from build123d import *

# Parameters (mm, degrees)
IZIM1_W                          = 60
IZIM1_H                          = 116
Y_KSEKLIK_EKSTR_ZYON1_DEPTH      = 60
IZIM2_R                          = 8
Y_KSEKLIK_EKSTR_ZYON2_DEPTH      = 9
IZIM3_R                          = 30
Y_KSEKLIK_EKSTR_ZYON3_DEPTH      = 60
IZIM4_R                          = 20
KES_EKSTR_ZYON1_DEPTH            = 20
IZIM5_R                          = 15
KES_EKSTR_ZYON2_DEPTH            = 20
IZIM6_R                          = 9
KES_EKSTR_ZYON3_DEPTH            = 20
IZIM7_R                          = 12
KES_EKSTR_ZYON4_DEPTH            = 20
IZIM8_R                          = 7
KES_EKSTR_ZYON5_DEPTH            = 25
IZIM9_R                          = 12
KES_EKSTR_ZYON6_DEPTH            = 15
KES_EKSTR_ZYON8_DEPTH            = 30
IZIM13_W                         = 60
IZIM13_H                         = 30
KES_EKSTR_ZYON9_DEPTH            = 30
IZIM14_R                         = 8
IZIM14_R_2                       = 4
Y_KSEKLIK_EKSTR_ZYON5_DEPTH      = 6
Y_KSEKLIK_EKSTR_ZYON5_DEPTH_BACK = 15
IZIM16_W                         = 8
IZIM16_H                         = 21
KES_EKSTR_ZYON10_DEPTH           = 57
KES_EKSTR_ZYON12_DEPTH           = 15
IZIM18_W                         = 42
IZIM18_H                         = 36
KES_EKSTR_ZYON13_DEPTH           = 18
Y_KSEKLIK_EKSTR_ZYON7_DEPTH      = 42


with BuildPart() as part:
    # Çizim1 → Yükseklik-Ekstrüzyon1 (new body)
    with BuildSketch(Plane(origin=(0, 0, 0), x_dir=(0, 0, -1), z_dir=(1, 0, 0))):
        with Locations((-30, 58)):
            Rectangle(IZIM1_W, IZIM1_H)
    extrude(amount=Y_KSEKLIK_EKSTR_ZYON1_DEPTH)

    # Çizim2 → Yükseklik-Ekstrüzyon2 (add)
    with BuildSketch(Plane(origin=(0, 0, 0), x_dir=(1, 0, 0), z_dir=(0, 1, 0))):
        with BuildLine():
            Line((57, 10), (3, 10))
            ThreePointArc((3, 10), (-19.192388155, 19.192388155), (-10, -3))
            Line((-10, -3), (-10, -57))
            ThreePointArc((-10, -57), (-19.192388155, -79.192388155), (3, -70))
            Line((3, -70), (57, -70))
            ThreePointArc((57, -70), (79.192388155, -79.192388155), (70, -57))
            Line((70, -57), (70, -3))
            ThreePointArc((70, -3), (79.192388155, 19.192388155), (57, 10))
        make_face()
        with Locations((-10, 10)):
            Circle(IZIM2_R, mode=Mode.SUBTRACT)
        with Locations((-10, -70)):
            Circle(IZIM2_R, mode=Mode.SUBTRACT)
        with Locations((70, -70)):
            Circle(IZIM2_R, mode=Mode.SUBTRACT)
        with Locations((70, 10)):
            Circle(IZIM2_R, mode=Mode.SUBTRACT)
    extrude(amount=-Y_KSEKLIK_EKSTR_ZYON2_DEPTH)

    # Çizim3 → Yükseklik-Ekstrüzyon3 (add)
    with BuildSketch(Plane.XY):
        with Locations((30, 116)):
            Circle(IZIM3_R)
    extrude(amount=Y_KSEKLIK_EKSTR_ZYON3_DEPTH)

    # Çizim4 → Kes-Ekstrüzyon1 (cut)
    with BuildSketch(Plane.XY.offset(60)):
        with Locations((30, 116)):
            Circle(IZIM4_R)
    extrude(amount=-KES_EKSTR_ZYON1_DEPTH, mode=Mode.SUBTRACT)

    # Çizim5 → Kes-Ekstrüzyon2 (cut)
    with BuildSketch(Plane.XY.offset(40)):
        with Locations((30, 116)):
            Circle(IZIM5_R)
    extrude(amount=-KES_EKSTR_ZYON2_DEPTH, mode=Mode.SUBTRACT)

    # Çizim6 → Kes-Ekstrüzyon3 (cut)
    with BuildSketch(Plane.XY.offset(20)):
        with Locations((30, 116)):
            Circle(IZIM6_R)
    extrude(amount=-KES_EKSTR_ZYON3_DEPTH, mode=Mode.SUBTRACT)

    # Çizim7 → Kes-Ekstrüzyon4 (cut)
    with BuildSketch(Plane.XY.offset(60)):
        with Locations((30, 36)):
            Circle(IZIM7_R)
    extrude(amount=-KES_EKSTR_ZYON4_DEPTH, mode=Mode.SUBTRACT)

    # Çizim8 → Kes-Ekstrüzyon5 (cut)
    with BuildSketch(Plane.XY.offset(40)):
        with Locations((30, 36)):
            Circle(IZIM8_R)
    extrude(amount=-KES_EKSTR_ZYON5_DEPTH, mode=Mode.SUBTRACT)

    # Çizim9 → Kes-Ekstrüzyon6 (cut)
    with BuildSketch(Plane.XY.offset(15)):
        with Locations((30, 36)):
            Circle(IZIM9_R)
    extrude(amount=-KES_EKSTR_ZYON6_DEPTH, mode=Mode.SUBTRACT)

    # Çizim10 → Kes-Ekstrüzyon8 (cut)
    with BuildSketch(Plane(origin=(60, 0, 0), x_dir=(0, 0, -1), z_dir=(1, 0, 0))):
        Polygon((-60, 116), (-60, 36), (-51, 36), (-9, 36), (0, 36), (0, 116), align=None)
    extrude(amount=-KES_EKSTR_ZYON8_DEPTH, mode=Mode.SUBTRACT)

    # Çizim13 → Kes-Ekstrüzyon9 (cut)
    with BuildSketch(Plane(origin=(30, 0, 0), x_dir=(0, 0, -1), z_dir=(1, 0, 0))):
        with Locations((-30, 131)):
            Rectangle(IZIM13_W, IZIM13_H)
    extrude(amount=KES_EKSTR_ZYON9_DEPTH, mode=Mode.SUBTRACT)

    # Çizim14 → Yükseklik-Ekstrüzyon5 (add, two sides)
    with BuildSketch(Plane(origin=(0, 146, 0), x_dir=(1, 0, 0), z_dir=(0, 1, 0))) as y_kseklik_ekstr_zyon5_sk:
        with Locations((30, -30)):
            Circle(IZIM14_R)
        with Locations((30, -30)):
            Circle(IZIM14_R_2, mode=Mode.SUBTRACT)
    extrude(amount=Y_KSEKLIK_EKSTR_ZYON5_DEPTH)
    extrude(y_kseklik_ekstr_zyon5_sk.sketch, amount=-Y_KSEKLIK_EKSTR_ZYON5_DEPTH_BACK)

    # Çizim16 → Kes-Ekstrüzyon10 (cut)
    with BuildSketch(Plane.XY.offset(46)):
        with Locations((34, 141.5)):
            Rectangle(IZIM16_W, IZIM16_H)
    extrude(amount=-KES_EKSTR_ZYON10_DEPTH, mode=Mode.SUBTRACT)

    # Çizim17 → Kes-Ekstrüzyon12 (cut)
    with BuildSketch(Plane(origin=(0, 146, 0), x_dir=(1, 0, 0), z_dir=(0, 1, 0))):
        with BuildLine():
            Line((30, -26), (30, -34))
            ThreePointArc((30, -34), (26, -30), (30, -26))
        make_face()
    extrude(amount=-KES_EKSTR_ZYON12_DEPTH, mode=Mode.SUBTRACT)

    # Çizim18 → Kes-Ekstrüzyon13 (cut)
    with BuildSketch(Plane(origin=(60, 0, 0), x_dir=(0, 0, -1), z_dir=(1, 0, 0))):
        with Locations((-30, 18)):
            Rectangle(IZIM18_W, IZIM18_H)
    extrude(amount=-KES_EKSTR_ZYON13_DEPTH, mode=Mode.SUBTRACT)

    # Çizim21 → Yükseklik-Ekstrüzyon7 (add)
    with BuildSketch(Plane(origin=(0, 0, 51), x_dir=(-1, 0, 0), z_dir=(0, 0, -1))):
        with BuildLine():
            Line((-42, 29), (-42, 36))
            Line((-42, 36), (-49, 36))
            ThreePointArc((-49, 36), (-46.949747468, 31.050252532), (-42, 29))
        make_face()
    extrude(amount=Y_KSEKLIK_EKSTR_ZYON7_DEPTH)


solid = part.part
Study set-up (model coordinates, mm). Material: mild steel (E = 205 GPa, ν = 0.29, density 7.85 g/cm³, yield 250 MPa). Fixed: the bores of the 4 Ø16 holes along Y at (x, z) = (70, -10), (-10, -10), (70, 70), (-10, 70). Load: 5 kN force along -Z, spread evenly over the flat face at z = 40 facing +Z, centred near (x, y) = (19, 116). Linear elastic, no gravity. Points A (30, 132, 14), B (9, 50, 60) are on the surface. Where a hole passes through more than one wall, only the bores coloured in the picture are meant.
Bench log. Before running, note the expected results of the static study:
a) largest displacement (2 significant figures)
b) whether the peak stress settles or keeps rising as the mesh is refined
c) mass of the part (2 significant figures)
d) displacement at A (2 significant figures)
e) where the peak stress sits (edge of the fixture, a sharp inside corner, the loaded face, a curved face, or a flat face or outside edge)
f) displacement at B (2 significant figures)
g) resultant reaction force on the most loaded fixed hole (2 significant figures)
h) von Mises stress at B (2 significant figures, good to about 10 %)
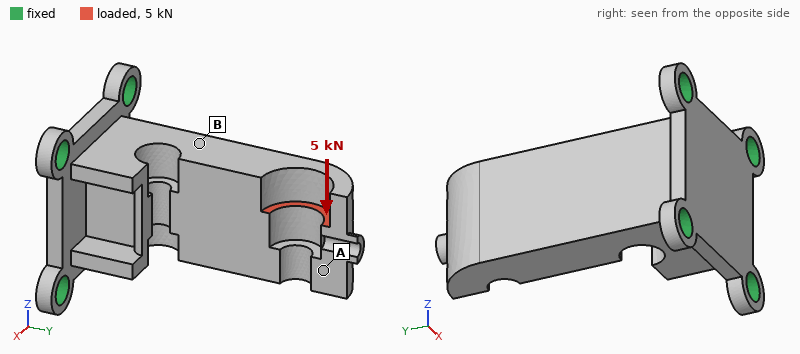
0.12 mm
keeps rising
2.5 kg
0.10 mm
edge of the fixture
0.037 mm
6.5 kN
26 MPa
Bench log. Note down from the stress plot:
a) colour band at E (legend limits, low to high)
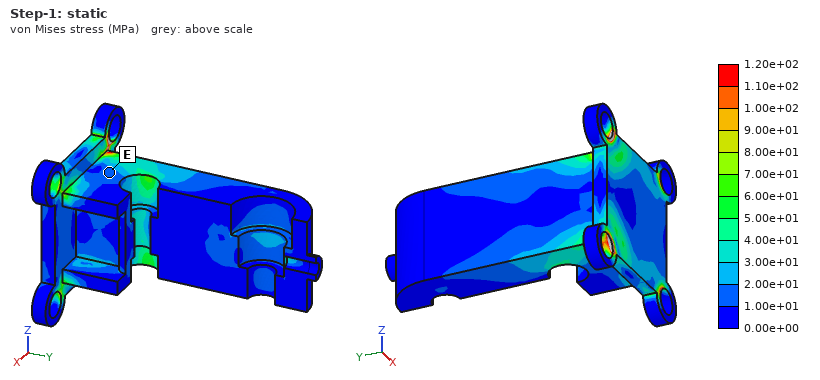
1.00e+01 to 2.00e+01 MPa
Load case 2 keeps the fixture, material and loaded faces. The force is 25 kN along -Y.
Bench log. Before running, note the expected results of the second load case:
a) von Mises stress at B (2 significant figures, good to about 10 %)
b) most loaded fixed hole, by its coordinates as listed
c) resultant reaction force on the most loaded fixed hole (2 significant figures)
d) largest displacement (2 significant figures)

38 MPa
(-10, 70)
12 kN
0.16 mm
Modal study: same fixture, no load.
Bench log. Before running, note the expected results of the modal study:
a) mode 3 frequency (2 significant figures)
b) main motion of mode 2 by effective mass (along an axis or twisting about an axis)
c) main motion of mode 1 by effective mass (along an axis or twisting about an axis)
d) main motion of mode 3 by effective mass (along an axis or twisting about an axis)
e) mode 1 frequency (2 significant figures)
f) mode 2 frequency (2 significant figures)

3600 Hz
along Z
along X
along Y
1000 Hz
1400 Hz
